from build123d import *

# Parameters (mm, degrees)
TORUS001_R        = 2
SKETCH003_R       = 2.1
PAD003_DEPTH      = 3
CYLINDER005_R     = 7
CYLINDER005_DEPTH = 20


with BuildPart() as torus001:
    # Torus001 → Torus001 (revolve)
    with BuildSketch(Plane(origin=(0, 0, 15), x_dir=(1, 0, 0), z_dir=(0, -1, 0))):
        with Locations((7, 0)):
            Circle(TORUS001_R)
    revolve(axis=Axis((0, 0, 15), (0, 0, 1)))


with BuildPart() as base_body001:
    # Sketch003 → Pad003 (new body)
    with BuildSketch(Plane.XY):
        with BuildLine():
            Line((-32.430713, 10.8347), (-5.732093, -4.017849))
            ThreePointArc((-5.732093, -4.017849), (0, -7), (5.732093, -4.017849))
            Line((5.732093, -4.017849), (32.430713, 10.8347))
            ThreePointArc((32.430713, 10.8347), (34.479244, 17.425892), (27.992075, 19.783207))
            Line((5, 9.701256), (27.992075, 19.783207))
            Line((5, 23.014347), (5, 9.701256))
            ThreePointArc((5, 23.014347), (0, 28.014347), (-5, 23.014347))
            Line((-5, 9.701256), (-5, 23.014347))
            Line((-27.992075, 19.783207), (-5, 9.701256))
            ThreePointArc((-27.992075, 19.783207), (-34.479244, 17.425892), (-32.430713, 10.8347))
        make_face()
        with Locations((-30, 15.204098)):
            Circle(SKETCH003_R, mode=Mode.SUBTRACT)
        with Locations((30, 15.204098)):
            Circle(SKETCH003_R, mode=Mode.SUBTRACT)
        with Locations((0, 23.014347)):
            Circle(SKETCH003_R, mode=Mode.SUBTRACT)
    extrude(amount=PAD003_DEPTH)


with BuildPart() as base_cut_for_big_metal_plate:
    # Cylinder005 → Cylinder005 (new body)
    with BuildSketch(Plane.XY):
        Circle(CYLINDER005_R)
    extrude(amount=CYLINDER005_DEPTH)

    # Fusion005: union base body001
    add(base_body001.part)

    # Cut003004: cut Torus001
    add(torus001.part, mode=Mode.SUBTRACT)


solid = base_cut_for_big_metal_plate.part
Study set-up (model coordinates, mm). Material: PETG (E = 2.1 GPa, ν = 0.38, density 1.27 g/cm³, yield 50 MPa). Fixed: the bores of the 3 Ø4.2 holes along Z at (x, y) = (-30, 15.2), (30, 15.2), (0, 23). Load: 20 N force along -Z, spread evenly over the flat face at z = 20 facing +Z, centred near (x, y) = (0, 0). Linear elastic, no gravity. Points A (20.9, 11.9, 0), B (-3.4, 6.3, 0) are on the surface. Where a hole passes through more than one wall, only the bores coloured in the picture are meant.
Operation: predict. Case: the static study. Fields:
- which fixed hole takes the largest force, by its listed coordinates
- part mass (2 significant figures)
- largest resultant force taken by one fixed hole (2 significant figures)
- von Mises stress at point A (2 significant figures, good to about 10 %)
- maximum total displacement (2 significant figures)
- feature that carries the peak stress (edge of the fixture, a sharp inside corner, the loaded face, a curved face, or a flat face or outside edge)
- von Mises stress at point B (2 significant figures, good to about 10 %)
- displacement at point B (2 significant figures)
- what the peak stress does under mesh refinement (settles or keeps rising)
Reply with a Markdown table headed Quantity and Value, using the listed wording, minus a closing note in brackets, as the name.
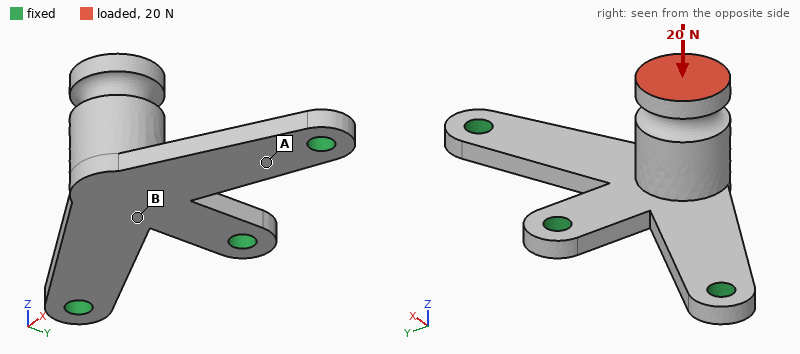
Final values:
| Quantity | Value |
|---|---|
| which fixed hole takes the largest force, by its listed coordinates | (0, 23) |
| part mass | 6.8 g |
| largest resultant force taken by one fixed hole | 8.8 N |
| von Mises stress at point A | 5.0 MPa |
| maximum total displacement | 0.80 mm |
| feature that carries the peak stress | edge of the fixture |
| von Mises stress at point B | 1.9 MPa |
| displacement at point B | 0.26 mm |
| what the peak stress does under mesh refinement | keeps rising |
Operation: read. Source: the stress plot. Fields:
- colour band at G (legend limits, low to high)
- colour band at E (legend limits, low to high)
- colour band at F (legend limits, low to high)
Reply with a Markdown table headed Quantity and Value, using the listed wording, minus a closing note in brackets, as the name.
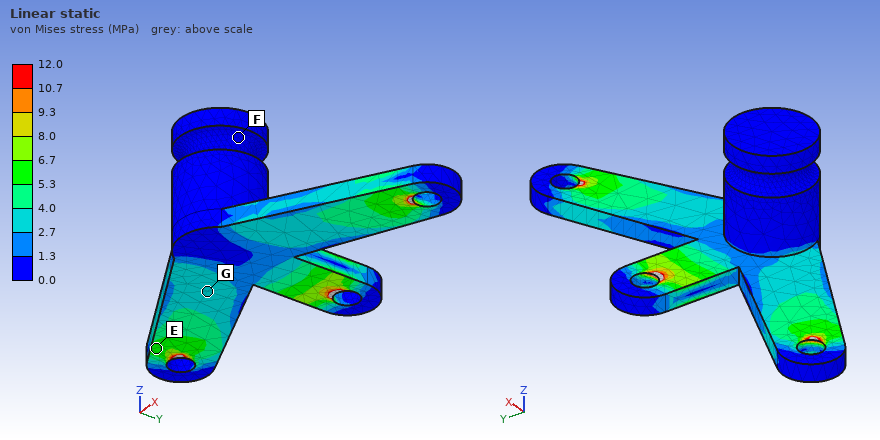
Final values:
| Quantity | Value |
|---|---|
| colour band at G | 2.7 to 4.0 MPa |
| colour band at E | 5.3 to 6.7 MPa |
| colour band at F | 0.0 to 1.3 MPa |
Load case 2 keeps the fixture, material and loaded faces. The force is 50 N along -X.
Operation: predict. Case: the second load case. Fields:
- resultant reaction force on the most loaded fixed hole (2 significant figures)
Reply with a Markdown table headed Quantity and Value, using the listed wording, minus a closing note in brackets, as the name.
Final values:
| Quantity | Value |
|---|---|
| resultant reaction force on the most loaded fixed hole | 33 N |
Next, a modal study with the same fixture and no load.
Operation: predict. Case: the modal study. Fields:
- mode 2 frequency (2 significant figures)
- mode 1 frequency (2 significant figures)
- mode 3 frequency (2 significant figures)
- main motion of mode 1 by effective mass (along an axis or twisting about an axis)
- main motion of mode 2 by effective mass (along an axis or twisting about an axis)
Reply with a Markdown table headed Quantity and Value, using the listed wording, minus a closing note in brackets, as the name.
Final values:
| Quantity | Value |
|---|---|
| mode 2 frequency | 1200 Hz |
| mode 1 frequency | 450 Hz |
| mode 3 frequency | 1700 Hz |
| main motion of mode 1 by effective mass | along Z |
| main motion of mode 2 by effective mass | along X |
